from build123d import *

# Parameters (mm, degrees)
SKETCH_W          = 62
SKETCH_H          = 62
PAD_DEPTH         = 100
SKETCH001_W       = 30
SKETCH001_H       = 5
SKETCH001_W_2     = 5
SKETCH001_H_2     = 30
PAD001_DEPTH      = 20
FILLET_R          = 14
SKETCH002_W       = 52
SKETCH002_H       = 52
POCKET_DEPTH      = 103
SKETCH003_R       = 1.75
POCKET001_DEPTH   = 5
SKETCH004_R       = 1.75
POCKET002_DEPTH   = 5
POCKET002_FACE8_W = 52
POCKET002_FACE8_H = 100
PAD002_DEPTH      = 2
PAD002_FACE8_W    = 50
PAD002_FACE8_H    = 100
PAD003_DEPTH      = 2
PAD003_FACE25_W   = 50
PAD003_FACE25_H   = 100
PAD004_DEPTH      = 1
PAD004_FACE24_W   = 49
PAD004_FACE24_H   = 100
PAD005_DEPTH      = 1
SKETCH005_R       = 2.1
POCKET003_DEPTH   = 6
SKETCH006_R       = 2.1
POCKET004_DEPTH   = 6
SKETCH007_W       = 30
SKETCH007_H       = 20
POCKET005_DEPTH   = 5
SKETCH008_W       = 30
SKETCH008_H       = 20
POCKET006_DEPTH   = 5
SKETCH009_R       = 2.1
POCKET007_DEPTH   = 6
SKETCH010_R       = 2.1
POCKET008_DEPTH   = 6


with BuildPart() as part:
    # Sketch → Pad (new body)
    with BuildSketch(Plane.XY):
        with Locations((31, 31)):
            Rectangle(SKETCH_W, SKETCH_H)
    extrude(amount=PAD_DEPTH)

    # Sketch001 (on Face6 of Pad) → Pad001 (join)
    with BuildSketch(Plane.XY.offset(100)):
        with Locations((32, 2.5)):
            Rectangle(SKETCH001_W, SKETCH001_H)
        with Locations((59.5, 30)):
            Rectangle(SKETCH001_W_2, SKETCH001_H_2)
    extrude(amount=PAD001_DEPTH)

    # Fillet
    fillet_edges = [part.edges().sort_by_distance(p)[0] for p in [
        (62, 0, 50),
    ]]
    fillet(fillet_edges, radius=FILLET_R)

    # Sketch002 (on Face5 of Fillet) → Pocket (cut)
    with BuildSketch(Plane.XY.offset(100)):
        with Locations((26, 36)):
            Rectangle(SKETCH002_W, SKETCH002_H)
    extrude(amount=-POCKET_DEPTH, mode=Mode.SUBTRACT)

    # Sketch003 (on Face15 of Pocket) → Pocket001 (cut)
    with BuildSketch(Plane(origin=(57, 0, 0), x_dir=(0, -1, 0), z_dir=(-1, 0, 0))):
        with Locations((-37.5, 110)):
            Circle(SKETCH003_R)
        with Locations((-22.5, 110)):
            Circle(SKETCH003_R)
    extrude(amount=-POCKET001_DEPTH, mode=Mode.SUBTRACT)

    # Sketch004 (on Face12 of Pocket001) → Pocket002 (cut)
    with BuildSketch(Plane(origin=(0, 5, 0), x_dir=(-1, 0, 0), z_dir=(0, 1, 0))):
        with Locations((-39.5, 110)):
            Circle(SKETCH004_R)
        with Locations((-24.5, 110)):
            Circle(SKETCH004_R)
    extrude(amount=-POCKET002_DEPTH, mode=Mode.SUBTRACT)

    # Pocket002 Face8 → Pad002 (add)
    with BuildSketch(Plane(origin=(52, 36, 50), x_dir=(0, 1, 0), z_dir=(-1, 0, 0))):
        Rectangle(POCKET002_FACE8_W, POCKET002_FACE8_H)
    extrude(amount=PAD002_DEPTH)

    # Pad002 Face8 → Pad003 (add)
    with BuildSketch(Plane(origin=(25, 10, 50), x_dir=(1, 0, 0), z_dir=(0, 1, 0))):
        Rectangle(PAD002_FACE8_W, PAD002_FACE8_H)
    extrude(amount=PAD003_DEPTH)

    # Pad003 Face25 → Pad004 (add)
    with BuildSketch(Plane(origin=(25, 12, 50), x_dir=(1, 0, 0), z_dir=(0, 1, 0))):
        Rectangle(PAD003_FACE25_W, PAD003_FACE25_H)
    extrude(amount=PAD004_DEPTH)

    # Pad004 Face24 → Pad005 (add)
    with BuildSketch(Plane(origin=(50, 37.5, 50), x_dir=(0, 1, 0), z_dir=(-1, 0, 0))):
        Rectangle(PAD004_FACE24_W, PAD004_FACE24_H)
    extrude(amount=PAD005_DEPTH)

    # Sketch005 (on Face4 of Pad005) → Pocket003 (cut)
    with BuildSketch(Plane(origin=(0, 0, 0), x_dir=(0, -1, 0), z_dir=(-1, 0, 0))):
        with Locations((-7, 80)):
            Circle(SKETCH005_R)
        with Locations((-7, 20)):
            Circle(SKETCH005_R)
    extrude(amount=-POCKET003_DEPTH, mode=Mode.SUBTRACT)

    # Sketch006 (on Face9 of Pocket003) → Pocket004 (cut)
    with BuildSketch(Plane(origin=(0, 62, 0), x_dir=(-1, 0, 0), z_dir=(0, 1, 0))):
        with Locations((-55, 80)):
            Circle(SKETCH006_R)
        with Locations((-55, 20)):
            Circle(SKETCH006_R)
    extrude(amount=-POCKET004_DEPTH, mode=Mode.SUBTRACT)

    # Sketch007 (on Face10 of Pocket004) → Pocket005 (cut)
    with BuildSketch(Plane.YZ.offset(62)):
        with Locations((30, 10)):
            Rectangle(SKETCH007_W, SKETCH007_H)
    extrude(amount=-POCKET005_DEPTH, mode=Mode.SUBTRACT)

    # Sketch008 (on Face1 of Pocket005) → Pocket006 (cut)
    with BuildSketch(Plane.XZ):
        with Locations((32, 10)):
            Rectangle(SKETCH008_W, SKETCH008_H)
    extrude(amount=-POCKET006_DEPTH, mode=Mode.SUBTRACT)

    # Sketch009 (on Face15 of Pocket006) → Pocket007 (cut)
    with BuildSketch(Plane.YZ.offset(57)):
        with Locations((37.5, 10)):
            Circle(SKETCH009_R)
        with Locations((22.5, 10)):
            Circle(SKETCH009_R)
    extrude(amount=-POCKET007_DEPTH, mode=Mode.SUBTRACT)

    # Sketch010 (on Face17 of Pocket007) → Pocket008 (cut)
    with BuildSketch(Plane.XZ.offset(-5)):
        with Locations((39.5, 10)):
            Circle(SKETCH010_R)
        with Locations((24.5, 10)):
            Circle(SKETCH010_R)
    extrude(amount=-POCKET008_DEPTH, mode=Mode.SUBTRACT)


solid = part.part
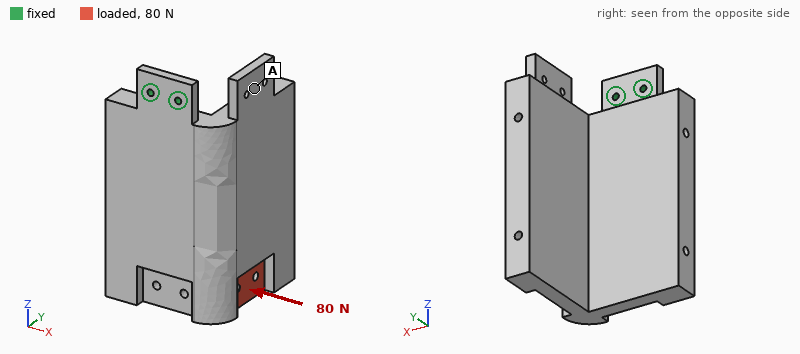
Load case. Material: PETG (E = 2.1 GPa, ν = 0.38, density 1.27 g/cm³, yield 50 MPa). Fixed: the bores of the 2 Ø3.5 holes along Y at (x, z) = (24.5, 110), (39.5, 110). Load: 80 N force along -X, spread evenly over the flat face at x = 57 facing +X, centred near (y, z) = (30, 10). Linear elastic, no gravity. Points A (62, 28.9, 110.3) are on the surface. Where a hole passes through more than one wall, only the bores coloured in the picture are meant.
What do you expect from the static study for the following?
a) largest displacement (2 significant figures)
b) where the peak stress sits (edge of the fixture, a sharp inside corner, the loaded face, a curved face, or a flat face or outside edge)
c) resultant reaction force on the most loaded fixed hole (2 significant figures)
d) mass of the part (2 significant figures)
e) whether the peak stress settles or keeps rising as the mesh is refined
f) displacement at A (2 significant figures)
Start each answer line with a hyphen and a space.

- 1.4 mm
- edge of the fixture
- 490 N
- 180 g
- keeps rising
- 0.35 mm
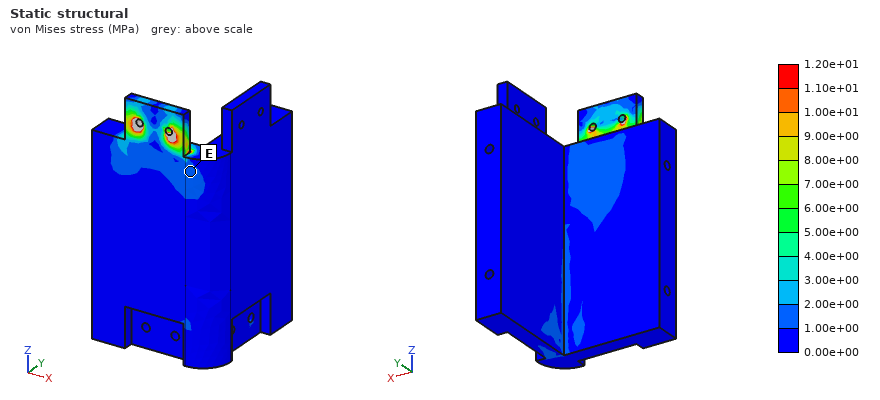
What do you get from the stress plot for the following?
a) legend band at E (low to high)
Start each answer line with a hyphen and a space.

- 1.00e+00 to 2.00e+00 MPa
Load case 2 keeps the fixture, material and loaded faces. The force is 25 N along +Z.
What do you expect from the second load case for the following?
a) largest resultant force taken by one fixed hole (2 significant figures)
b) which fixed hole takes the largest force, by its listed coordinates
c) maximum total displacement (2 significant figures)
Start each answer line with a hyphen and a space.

- 50 N
- (39.5, 110)
- 1.5 mm
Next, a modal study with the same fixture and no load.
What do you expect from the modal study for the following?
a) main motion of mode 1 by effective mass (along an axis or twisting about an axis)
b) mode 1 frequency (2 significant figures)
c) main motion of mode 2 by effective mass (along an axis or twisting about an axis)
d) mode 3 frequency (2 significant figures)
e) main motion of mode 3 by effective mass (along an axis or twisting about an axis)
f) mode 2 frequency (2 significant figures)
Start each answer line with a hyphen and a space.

- along Y
- 44 Hz
- along X
- 230 Hz
- along X
- 150 Hz
